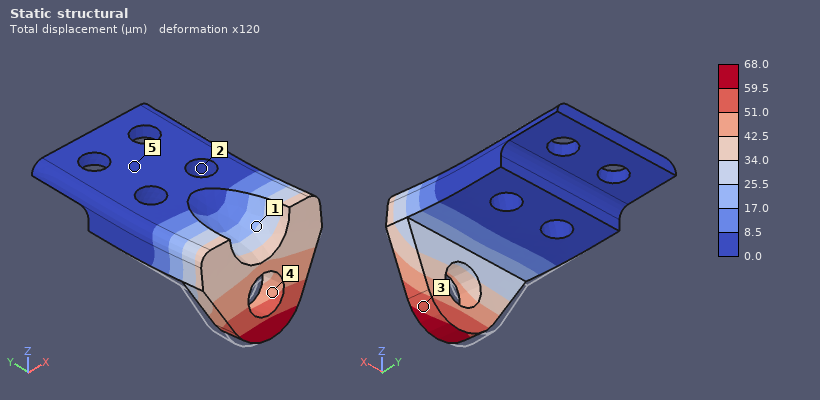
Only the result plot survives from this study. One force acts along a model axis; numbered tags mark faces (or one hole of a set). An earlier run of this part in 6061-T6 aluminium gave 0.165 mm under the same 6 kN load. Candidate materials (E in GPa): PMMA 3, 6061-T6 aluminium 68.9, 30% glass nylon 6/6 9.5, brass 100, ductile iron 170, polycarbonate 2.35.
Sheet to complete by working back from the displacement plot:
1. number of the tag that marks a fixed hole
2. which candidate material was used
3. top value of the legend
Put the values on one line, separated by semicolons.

2; ductile iron; 68.0 µm
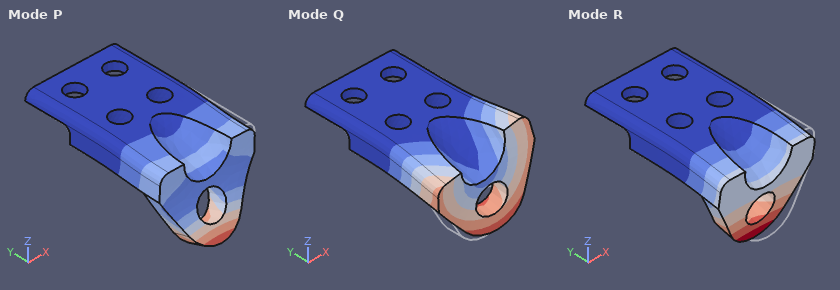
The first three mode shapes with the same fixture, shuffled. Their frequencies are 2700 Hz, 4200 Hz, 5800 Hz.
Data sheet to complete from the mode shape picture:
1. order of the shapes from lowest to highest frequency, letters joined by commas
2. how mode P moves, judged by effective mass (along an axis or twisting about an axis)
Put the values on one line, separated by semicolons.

R, Q, P; along Z
